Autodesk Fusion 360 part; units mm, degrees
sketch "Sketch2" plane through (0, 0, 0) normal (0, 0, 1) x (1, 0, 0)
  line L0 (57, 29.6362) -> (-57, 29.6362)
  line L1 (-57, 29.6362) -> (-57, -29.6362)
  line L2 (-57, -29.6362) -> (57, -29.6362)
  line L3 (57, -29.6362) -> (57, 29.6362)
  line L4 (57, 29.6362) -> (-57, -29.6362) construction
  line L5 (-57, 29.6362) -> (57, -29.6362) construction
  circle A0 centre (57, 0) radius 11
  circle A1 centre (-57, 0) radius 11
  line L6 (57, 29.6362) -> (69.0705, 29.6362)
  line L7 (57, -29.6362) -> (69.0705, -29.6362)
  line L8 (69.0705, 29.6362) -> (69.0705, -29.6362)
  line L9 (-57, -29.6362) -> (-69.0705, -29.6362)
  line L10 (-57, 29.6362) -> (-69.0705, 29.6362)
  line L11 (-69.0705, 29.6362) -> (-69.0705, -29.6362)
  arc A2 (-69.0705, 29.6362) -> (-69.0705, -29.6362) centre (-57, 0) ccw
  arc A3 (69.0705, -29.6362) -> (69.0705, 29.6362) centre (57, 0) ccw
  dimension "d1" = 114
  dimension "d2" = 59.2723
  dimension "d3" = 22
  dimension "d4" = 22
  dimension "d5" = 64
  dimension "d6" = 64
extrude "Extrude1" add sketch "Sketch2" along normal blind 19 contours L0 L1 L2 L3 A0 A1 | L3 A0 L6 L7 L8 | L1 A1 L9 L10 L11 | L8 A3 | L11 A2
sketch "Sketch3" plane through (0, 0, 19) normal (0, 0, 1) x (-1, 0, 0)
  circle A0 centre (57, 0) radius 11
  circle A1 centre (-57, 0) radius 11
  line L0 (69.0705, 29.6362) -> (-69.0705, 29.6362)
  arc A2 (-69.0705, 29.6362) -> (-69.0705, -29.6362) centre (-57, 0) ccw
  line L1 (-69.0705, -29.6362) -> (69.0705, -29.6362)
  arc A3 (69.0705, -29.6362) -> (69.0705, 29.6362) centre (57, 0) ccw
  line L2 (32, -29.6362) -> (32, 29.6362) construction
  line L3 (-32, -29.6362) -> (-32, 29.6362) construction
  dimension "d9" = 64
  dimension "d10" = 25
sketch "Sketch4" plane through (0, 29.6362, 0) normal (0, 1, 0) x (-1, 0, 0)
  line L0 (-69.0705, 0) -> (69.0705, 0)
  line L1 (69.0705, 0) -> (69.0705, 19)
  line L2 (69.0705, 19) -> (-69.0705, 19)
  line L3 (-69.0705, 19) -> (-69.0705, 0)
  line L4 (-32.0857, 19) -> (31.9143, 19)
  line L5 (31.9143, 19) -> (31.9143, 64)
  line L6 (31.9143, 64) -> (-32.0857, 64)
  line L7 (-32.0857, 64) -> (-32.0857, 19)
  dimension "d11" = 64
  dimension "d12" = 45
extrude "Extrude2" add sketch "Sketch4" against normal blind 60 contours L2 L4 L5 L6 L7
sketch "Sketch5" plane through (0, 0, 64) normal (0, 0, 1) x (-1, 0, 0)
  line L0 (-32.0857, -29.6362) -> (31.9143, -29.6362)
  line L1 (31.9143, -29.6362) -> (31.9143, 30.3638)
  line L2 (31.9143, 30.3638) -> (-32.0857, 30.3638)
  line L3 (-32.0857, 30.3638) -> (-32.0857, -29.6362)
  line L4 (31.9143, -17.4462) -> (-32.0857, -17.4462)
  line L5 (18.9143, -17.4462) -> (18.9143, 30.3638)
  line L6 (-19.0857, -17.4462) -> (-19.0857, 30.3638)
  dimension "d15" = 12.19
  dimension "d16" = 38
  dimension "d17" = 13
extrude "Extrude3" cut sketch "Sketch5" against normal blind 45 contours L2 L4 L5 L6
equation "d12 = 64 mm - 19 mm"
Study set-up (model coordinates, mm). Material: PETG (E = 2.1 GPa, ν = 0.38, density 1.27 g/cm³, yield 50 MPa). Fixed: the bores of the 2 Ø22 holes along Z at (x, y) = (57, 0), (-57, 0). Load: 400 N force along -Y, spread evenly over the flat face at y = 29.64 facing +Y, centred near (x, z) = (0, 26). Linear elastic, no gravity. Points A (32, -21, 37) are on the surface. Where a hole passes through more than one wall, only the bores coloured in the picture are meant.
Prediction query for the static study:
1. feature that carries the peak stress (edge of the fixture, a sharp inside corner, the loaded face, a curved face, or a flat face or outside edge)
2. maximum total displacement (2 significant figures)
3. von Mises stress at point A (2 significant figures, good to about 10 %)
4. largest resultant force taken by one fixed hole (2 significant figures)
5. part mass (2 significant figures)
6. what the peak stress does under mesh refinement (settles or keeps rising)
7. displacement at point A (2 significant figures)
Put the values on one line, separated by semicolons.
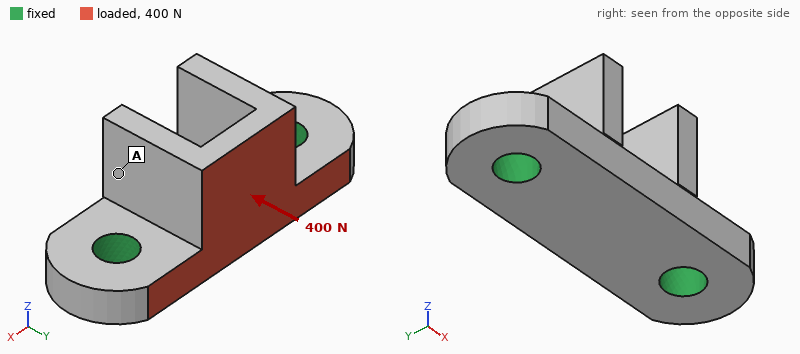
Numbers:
edge of the fixture; 68 µm; 0.20 MPa; 200 N; 340 g; keeps rising; 33 µm
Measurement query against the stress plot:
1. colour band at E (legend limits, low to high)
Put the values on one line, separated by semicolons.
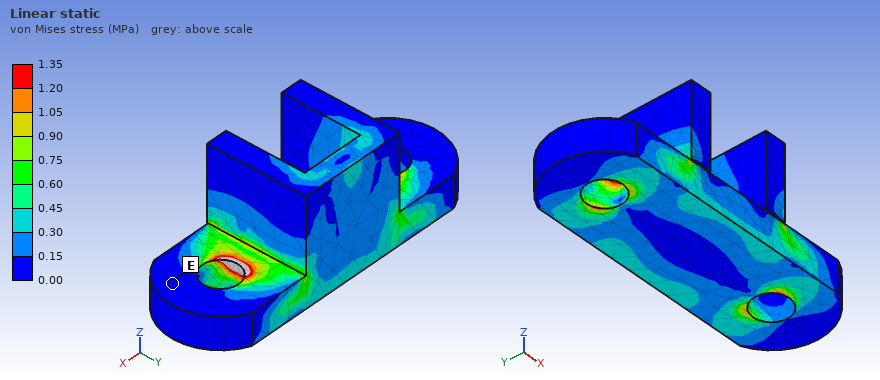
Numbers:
0.00 to 0.15 MPa
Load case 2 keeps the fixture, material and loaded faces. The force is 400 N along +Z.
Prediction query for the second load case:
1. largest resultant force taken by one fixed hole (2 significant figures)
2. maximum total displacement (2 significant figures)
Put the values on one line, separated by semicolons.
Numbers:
210 N; 83 µm
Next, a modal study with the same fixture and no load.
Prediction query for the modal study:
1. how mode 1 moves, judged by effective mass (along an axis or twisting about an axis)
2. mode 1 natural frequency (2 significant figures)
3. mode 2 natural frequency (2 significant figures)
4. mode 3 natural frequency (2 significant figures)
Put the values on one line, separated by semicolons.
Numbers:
along Y; 970 Hz; 1400 Hz; 1400 Hz
